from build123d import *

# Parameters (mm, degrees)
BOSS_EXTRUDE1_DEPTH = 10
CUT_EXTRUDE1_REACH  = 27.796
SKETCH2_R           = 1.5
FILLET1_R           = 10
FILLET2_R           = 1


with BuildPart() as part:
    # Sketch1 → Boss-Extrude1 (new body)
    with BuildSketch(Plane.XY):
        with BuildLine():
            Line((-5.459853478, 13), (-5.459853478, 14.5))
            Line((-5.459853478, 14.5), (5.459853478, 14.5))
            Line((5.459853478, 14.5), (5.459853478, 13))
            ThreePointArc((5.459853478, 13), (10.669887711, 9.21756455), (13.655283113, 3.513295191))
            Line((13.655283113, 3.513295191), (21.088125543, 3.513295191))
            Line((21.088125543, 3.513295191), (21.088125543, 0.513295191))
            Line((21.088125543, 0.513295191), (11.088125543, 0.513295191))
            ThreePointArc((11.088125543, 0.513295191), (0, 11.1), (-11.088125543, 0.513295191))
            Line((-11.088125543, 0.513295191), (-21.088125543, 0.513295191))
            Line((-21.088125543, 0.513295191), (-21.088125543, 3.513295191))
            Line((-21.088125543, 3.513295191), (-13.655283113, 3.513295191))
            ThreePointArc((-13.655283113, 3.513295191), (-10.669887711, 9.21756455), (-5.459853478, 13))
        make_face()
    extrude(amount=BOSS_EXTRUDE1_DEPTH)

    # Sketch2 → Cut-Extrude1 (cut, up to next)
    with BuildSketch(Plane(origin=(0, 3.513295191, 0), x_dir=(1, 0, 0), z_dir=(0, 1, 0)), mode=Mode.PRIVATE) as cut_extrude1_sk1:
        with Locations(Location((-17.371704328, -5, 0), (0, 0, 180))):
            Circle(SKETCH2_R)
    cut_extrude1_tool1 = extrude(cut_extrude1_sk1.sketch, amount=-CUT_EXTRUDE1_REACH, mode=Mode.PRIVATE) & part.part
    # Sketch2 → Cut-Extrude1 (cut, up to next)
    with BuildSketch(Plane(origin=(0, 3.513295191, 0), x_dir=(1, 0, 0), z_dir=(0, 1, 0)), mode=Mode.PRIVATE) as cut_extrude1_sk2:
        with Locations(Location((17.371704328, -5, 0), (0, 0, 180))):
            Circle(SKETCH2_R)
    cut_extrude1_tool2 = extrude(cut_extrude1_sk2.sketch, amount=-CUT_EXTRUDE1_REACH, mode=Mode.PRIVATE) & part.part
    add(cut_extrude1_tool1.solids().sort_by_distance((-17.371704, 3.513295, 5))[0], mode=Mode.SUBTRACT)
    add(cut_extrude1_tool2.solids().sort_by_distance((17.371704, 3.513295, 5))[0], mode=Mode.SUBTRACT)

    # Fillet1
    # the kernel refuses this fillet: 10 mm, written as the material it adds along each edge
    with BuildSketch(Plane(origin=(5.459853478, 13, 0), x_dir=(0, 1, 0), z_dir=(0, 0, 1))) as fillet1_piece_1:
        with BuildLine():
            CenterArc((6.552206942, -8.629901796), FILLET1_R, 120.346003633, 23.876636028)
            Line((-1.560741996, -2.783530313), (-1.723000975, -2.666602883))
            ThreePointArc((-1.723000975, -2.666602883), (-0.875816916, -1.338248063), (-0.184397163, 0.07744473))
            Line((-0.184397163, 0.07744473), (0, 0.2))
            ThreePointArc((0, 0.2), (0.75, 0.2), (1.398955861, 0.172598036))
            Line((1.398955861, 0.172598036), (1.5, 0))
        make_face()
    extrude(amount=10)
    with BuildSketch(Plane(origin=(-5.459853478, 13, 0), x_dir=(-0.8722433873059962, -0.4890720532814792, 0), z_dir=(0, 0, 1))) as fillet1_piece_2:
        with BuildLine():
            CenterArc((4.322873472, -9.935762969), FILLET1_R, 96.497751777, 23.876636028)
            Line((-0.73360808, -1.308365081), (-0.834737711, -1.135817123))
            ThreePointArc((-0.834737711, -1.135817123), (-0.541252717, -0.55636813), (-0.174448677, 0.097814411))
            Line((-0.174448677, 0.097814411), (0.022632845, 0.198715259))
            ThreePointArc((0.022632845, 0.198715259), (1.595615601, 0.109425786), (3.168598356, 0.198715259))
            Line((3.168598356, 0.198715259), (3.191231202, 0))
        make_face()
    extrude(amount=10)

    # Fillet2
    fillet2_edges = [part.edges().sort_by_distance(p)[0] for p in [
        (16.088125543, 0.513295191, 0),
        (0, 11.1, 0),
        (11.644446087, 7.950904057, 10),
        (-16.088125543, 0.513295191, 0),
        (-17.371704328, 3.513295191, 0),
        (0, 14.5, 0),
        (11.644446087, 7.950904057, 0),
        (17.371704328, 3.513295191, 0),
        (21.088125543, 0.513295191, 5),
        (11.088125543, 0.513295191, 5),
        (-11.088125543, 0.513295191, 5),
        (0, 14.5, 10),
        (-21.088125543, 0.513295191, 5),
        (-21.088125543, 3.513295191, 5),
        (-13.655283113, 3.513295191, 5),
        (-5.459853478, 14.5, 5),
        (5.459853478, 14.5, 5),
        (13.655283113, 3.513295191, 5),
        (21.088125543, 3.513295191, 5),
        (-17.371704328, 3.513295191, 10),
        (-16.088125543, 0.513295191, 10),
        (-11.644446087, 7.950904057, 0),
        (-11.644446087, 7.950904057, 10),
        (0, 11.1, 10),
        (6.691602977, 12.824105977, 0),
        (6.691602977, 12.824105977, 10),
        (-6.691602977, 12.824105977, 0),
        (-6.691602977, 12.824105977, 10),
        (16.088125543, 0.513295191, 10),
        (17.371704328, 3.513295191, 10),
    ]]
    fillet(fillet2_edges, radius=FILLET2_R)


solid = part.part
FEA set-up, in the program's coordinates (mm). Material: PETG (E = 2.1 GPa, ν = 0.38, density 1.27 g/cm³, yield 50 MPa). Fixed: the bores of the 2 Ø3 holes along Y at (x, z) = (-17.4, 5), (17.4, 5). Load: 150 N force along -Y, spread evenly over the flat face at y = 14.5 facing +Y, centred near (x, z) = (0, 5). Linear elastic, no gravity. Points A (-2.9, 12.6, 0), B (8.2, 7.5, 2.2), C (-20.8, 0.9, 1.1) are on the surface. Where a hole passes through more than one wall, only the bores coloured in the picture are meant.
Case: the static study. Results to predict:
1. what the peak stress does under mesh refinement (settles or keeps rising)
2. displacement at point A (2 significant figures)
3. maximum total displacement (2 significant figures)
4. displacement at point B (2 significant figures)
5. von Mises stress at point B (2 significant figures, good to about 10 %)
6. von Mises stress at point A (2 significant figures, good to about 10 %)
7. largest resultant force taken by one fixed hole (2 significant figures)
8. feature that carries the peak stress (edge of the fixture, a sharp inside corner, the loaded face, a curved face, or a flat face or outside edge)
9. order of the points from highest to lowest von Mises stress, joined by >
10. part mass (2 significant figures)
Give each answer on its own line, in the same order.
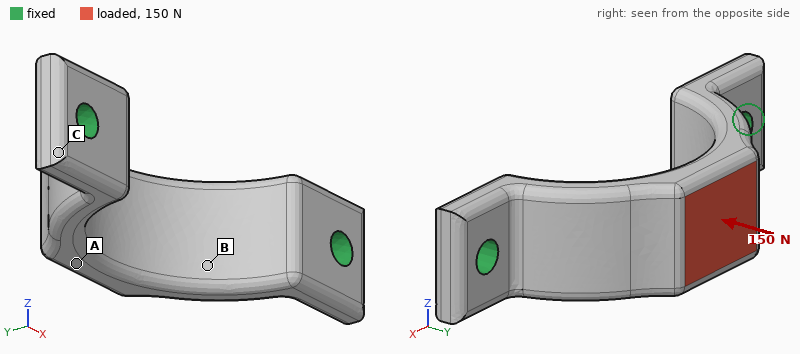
keeps rising
80 µm
90 µm
40 µm
8.0 MPa
4.2 MPa
100 N
edge of the fixture
B > A > C
2.0 g
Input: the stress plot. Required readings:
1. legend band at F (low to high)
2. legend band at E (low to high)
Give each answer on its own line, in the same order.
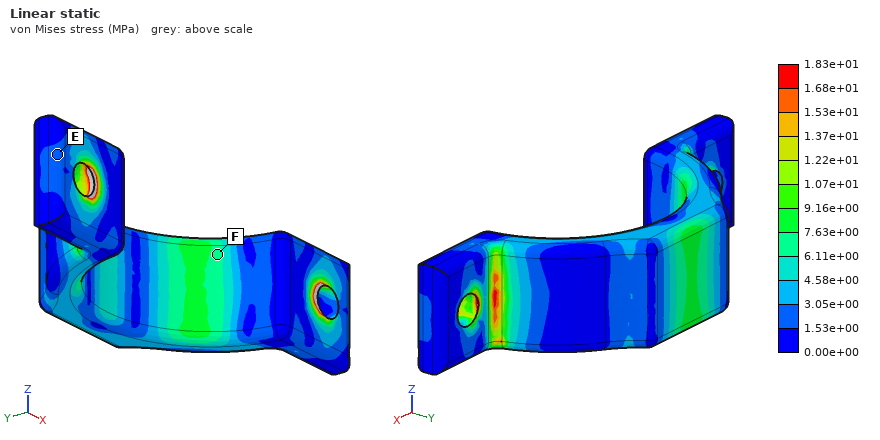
6.11e+00 to 7.63e+00 MPa
1.53e+00 to 3.05e+00 MPa
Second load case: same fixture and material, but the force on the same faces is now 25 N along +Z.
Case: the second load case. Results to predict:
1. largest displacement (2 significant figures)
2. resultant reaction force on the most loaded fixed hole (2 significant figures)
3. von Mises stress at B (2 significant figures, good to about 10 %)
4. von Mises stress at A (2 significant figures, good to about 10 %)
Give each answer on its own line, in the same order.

0.17 mm
13 N
1.5 MPa
0.99 MPa
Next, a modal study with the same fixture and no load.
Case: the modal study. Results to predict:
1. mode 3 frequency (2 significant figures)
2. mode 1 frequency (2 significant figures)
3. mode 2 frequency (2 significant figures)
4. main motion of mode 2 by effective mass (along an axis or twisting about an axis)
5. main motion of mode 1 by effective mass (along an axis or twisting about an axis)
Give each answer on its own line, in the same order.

7200 Hz
2400 Hz
4800 Hz
along X
along Z
